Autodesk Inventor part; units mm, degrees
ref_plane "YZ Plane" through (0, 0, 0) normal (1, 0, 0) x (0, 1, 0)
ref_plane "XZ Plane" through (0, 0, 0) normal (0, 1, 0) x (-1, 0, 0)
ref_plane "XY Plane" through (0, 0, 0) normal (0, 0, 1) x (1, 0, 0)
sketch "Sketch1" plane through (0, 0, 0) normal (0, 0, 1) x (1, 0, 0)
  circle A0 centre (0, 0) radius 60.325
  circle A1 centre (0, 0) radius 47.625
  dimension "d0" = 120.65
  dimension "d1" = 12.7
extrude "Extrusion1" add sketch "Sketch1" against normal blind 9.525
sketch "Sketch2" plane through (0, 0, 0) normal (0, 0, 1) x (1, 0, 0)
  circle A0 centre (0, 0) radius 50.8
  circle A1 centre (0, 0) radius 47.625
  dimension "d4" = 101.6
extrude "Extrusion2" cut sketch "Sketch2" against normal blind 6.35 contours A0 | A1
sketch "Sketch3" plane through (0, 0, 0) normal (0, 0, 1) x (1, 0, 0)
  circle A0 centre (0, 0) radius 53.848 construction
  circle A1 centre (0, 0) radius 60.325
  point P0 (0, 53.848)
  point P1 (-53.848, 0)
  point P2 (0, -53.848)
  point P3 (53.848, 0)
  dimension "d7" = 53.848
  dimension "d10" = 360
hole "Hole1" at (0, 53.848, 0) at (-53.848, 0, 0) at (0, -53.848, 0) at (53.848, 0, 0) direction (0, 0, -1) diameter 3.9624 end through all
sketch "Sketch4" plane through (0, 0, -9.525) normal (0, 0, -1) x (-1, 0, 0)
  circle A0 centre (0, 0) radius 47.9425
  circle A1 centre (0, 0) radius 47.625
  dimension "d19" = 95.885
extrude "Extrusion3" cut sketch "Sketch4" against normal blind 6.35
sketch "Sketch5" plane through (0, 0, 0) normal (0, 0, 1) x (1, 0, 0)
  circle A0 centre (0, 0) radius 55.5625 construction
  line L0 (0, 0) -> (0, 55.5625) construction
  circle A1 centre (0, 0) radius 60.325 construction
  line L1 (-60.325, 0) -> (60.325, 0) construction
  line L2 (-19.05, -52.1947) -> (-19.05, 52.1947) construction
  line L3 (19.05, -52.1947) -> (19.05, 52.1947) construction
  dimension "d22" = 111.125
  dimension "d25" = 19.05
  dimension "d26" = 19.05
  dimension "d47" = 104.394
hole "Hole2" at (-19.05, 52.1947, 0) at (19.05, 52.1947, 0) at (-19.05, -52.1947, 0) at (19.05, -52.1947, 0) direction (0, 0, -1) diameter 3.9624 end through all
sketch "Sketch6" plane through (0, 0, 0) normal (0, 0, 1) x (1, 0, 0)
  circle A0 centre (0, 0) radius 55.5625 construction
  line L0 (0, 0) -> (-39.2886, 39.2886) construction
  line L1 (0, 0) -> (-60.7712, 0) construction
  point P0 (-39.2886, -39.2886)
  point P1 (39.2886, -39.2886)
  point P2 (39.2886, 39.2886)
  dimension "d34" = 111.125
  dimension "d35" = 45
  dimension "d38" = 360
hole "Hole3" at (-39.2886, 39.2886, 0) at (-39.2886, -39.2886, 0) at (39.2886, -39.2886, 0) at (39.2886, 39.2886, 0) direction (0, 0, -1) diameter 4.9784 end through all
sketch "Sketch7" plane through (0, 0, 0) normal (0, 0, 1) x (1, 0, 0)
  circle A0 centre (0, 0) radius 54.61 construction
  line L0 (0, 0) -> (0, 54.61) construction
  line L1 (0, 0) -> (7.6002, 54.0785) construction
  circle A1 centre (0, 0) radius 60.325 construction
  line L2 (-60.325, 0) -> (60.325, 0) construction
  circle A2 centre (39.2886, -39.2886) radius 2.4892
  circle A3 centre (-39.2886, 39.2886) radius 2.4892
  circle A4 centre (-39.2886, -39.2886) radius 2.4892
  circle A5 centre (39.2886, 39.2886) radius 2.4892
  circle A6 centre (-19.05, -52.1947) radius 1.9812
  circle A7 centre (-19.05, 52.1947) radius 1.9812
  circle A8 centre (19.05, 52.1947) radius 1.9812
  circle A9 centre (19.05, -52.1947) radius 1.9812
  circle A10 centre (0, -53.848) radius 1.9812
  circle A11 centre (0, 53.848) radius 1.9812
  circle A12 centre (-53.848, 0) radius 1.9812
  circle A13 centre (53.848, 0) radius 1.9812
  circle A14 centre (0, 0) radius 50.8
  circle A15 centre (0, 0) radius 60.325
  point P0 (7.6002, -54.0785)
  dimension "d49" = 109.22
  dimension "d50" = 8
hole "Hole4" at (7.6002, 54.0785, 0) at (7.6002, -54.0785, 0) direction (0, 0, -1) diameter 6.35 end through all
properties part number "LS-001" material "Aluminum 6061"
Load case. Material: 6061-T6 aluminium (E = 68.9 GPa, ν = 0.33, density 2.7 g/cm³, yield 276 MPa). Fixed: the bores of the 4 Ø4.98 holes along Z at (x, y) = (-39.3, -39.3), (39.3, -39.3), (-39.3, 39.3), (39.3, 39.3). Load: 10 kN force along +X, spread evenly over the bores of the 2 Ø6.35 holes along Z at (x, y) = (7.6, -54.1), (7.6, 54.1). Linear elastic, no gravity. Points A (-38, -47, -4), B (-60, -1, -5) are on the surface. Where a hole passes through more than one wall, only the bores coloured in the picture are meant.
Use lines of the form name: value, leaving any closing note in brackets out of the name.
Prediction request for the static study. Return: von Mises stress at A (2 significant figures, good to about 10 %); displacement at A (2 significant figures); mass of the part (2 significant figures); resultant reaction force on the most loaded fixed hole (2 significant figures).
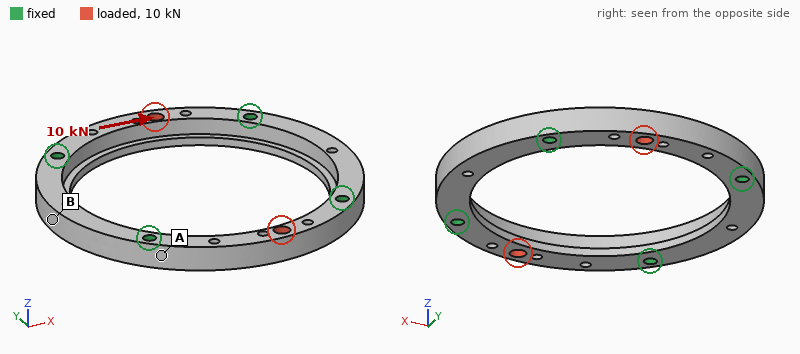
von Mises stress at A: 38 MPa
displacement at A: 7.4 µm
mass of the part: 87 g
resultant reaction force on the most loaded fixed hole: 2.7 kN
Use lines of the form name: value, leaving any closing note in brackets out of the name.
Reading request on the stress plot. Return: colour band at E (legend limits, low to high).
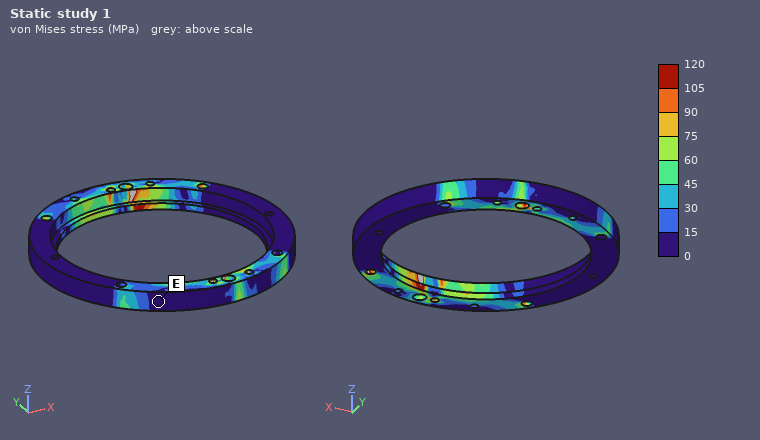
colour band at E: 0 to 15 MPa
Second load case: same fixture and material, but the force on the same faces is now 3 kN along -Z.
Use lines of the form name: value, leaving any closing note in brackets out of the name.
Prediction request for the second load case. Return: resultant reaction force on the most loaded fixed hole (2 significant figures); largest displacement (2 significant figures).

resultant reaction force on the most loaded fixed hole: 1.0 kN
largest displacement: 0.15 mm
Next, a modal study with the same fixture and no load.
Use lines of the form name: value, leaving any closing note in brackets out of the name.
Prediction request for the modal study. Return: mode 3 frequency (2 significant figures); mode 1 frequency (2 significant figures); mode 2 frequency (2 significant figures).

mode 3 frequency: 6100 Hz
mode 1 frequency: 5900 Hz
mode 2 frequency: 5900 Hz
